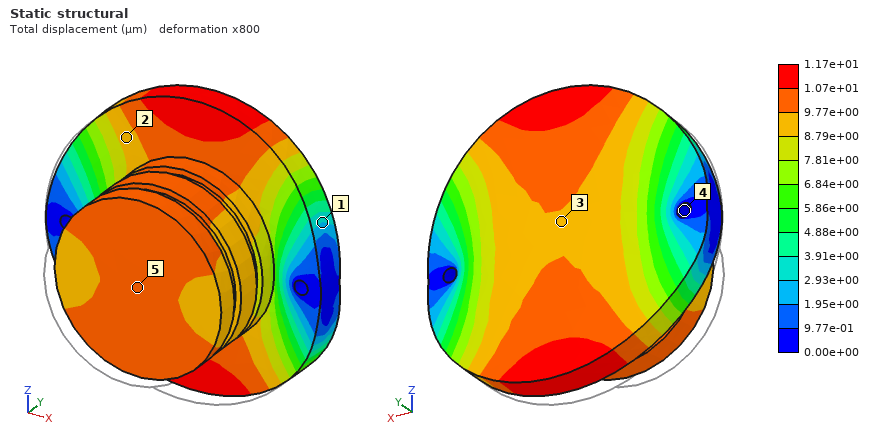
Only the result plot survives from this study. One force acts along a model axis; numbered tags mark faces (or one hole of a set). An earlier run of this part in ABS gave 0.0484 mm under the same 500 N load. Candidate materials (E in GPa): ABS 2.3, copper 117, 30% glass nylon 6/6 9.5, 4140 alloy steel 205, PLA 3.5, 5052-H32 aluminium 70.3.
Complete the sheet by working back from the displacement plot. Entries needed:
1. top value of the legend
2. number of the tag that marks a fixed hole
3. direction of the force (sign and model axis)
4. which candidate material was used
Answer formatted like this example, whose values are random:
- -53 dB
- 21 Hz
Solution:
- 1.17e+01 µm
- 4
- +Y
- 30% glass nylon 6/6
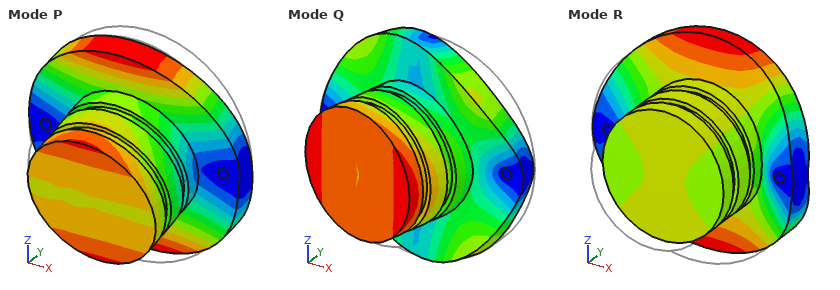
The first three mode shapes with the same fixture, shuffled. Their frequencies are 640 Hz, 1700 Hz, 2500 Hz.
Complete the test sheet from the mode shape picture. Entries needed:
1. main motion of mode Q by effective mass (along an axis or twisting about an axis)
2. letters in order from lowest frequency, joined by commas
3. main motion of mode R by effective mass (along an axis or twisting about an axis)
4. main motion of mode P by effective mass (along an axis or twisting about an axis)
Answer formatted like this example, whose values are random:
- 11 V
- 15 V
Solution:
- along X
- P, R, Q
- along Y
- along Z
